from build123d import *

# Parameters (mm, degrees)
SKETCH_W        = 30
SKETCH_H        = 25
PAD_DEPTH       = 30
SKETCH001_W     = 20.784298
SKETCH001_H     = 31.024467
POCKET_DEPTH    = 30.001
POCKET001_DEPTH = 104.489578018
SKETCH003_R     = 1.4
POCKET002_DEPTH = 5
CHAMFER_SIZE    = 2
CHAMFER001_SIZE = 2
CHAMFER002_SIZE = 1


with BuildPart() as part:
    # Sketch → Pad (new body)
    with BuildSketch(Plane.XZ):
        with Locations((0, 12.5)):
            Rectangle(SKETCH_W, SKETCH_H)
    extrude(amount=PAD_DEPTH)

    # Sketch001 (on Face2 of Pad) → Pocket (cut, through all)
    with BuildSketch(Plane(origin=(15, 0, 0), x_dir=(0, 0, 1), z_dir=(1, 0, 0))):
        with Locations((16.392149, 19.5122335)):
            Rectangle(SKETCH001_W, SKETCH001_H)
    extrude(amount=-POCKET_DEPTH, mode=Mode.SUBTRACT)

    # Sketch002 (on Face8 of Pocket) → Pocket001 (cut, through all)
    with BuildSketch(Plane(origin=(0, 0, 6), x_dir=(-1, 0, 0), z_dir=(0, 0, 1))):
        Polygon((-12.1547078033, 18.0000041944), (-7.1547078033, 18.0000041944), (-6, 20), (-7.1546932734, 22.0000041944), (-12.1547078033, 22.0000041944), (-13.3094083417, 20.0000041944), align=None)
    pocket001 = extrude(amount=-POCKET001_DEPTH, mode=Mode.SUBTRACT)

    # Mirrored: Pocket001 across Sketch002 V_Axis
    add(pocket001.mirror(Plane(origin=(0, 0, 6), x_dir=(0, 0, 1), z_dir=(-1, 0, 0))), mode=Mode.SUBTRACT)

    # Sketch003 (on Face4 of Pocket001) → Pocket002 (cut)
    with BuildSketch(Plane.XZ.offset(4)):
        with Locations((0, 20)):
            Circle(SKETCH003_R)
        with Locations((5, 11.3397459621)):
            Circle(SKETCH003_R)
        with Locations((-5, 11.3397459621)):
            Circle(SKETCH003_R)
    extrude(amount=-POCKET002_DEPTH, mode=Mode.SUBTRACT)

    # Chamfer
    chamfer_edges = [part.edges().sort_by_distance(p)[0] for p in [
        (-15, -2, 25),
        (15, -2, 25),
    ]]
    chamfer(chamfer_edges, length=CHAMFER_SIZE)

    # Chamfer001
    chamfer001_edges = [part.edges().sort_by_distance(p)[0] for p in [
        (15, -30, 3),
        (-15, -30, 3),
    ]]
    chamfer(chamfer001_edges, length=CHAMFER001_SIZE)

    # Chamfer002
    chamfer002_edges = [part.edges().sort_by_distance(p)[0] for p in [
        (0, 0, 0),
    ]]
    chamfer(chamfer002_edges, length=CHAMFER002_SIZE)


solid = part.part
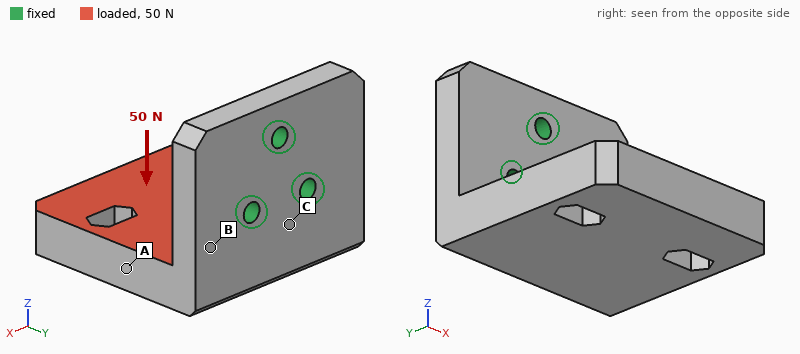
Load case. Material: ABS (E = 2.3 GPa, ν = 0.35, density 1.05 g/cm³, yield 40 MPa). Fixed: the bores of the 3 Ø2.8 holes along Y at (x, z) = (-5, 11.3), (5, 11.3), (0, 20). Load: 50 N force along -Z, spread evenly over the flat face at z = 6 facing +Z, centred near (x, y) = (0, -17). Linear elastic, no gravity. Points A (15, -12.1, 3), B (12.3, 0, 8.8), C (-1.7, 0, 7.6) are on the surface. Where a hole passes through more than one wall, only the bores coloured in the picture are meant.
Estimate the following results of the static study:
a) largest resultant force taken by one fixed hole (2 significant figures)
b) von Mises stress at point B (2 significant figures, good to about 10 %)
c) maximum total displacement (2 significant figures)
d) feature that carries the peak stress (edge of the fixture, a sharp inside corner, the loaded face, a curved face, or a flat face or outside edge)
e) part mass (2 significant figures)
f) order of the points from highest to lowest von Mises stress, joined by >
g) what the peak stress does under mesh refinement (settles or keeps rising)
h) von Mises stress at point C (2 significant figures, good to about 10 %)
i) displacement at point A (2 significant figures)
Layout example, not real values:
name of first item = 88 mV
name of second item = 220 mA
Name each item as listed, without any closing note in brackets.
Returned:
largest resultant force taken by one fixed hole = 25 N
von Mises stress at point B = 6.0 MPa
maximum total displacement = 0.53 mm
feature that carries the peak stress = edge of the fixture
part mass = 7.6 g
order of the points from highest to lowest von Mises stress, joined by > = C > B > A
what the peak stress does under mesh refinement = keeps rising
von Mises stress at point C = 8.3 MPa
displacement at point A = 0.18 mm
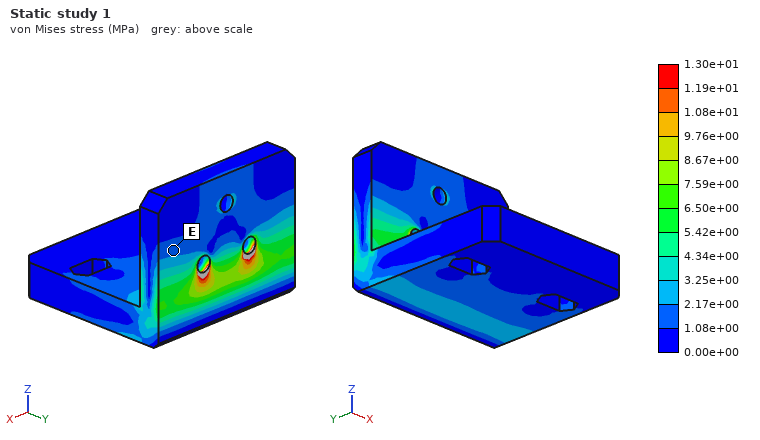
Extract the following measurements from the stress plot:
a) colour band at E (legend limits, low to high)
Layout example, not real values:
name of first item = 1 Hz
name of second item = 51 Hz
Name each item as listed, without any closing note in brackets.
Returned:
colour band at E = 1.08e+00 to 2.17e+00 MPa
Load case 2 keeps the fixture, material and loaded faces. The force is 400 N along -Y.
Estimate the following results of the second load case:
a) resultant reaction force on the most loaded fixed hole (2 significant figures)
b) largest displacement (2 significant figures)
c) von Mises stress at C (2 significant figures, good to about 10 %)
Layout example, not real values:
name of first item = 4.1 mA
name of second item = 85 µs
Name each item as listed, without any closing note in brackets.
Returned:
resultant reaction force on the most loaded fixed hole = 220 N
largest displacement = 0.28 mm
von Mises stress at C = 7.5 MPa
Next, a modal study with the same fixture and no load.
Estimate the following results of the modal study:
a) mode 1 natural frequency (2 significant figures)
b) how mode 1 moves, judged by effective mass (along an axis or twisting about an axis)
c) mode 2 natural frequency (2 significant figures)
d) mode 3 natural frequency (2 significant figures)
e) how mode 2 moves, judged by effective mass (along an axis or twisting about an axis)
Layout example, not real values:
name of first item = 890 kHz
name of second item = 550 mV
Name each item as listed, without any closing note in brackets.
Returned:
mode 1 natural frequency = 870 Hz
how mode 1 moves, judged by effective mass = along Z
mode 2 natural frequency = 1600 Hz
mode 3 natural frequency = 3200 Hz
how mode 2 moves, judged by effective mass = along X
